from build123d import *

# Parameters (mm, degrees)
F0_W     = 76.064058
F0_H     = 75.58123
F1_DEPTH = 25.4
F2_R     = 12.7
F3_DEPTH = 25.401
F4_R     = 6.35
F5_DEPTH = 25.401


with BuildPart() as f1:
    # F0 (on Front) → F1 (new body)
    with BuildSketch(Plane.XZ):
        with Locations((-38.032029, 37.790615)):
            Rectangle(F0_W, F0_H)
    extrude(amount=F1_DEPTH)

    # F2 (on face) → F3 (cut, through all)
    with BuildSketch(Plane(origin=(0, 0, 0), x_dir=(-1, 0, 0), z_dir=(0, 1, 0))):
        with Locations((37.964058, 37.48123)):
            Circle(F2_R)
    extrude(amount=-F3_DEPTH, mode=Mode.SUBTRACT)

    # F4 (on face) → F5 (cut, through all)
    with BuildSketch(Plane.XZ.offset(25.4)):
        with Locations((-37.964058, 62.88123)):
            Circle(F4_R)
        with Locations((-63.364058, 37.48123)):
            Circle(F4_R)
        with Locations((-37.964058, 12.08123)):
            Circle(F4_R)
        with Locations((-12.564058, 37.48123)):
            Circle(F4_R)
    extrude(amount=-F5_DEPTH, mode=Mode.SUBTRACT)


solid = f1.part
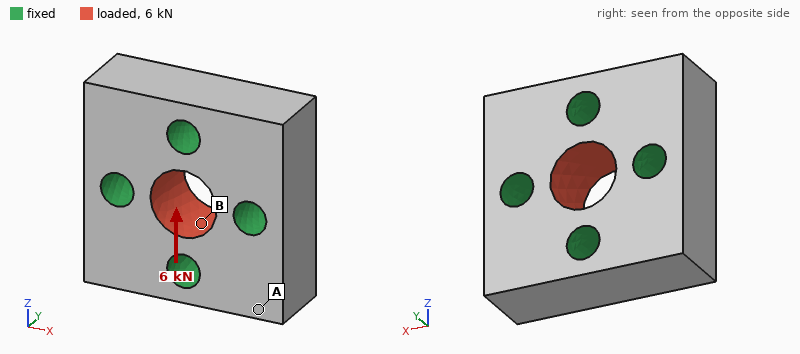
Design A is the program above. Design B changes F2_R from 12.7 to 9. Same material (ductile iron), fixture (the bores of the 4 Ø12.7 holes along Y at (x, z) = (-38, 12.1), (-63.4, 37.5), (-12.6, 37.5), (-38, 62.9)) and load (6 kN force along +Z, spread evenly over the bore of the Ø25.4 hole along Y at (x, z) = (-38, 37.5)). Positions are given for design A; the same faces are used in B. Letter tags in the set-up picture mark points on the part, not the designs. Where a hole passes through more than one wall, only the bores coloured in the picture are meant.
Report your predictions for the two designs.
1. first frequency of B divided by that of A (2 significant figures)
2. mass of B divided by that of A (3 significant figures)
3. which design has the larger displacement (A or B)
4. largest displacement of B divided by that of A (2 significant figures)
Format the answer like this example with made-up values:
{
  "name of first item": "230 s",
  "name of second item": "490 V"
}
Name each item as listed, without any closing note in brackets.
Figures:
{
  "first frequency of B divided by that of A": "1.0",
  "mass of B divided by that of A": "1.05",
  "which design has the larger displacement": "B",
  "largest displacement of B divided by that of A": "1.4"
}
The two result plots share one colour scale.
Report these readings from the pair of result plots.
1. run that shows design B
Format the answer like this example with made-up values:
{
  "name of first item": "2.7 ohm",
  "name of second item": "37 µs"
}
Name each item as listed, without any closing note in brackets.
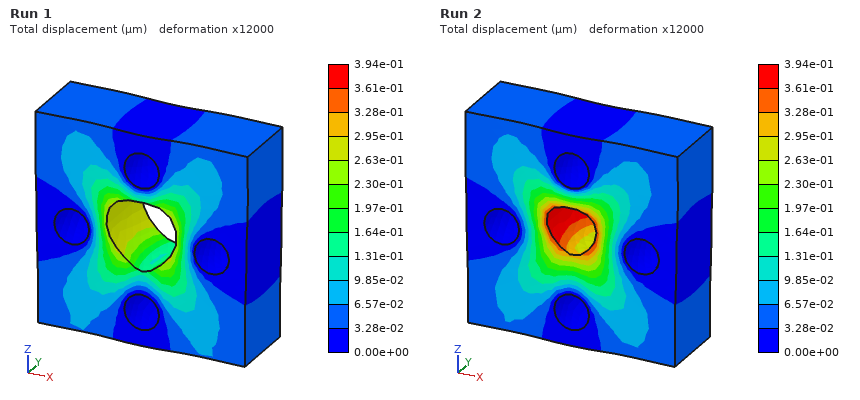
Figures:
{
  "run that shows design B": "Run 2"
}
